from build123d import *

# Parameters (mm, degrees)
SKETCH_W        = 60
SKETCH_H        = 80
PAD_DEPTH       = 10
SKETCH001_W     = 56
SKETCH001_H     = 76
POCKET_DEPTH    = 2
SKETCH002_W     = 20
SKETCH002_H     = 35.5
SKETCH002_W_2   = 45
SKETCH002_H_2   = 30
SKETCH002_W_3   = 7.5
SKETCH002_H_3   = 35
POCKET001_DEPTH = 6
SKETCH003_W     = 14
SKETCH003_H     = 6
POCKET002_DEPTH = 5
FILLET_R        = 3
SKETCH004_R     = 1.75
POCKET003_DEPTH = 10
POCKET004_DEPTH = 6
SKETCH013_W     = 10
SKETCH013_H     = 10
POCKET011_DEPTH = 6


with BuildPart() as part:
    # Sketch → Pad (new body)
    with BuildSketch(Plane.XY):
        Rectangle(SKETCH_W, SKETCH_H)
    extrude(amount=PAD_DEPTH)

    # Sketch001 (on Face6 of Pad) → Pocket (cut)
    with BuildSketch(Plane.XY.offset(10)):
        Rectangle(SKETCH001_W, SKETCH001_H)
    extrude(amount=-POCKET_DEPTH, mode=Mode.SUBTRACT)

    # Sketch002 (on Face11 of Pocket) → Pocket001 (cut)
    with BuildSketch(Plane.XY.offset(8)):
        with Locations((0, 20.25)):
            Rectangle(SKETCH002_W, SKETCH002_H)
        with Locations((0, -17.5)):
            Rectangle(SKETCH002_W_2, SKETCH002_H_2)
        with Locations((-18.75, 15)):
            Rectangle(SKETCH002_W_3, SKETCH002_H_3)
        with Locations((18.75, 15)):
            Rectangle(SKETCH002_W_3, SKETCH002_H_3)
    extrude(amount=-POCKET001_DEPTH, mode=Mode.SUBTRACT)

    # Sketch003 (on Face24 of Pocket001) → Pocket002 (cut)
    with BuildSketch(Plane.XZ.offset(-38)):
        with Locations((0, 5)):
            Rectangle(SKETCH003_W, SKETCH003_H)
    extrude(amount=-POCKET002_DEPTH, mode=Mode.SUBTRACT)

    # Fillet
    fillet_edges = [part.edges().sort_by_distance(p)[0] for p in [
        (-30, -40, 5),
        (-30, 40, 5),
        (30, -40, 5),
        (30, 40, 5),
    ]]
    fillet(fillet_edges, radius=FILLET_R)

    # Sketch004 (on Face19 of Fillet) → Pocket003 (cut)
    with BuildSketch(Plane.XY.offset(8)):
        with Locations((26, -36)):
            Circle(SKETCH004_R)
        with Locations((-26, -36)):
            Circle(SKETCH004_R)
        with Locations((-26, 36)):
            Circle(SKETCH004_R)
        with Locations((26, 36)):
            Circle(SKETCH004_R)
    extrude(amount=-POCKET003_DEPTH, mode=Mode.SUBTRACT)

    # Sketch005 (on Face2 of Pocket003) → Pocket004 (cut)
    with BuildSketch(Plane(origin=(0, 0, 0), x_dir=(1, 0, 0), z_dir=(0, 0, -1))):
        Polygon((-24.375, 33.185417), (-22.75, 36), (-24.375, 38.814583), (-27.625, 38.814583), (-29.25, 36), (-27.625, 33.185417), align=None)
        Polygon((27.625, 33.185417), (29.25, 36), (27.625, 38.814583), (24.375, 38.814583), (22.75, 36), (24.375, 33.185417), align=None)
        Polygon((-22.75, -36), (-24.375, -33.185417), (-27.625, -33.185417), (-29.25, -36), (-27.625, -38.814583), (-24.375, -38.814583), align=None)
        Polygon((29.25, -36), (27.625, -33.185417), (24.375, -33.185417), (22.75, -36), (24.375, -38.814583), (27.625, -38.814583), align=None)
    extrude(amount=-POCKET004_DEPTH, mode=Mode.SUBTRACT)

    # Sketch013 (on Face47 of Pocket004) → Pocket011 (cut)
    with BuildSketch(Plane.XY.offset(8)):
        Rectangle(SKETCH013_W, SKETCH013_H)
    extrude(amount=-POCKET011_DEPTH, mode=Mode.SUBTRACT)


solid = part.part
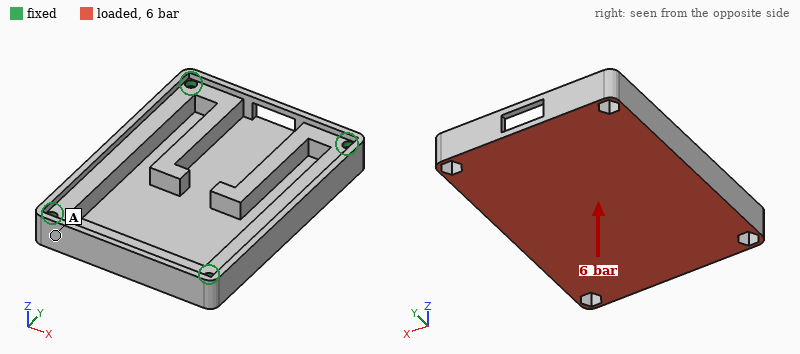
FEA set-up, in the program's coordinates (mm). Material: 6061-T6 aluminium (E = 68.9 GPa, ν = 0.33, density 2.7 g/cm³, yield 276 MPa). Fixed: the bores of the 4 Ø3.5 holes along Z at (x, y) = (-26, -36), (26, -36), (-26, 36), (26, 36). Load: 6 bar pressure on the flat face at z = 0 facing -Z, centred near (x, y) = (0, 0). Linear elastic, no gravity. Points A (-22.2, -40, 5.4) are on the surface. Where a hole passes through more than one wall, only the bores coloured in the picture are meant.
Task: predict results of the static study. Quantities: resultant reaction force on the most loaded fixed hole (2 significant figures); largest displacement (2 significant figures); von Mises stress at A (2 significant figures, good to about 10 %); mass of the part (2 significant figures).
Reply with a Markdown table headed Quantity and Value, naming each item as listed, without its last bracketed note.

| Quantity | Value |
|---|---|
| resultant reaction force on the most loaded fixed hole | 1.5 kN |
| largest displacement | 0.17 mm |
| von Mises stress at A | 18 MPa |
| mass of the part | 61 g |
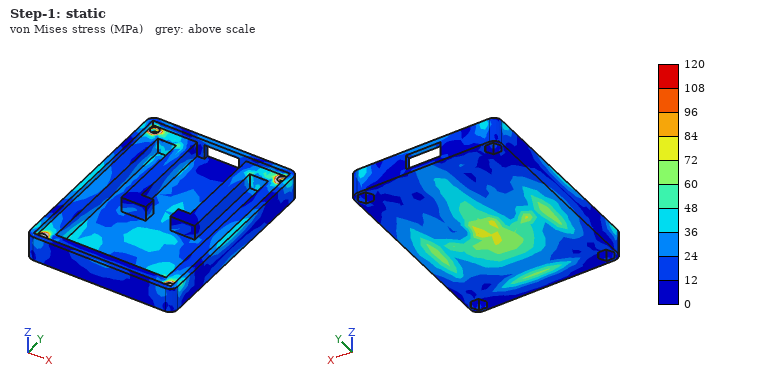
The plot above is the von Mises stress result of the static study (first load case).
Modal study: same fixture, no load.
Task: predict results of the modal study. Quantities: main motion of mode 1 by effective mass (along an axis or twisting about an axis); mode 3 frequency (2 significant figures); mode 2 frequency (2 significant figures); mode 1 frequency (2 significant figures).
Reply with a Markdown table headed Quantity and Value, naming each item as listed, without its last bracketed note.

| Quantity | Value |
|---|---|
| main motion of mode 1 by effective mass | along Z |
| mode 3 frequency | 7200 Hz |
| mode 2 frequency | 5600 Hz |
| mode 1 frequency | 4300 Hz |
